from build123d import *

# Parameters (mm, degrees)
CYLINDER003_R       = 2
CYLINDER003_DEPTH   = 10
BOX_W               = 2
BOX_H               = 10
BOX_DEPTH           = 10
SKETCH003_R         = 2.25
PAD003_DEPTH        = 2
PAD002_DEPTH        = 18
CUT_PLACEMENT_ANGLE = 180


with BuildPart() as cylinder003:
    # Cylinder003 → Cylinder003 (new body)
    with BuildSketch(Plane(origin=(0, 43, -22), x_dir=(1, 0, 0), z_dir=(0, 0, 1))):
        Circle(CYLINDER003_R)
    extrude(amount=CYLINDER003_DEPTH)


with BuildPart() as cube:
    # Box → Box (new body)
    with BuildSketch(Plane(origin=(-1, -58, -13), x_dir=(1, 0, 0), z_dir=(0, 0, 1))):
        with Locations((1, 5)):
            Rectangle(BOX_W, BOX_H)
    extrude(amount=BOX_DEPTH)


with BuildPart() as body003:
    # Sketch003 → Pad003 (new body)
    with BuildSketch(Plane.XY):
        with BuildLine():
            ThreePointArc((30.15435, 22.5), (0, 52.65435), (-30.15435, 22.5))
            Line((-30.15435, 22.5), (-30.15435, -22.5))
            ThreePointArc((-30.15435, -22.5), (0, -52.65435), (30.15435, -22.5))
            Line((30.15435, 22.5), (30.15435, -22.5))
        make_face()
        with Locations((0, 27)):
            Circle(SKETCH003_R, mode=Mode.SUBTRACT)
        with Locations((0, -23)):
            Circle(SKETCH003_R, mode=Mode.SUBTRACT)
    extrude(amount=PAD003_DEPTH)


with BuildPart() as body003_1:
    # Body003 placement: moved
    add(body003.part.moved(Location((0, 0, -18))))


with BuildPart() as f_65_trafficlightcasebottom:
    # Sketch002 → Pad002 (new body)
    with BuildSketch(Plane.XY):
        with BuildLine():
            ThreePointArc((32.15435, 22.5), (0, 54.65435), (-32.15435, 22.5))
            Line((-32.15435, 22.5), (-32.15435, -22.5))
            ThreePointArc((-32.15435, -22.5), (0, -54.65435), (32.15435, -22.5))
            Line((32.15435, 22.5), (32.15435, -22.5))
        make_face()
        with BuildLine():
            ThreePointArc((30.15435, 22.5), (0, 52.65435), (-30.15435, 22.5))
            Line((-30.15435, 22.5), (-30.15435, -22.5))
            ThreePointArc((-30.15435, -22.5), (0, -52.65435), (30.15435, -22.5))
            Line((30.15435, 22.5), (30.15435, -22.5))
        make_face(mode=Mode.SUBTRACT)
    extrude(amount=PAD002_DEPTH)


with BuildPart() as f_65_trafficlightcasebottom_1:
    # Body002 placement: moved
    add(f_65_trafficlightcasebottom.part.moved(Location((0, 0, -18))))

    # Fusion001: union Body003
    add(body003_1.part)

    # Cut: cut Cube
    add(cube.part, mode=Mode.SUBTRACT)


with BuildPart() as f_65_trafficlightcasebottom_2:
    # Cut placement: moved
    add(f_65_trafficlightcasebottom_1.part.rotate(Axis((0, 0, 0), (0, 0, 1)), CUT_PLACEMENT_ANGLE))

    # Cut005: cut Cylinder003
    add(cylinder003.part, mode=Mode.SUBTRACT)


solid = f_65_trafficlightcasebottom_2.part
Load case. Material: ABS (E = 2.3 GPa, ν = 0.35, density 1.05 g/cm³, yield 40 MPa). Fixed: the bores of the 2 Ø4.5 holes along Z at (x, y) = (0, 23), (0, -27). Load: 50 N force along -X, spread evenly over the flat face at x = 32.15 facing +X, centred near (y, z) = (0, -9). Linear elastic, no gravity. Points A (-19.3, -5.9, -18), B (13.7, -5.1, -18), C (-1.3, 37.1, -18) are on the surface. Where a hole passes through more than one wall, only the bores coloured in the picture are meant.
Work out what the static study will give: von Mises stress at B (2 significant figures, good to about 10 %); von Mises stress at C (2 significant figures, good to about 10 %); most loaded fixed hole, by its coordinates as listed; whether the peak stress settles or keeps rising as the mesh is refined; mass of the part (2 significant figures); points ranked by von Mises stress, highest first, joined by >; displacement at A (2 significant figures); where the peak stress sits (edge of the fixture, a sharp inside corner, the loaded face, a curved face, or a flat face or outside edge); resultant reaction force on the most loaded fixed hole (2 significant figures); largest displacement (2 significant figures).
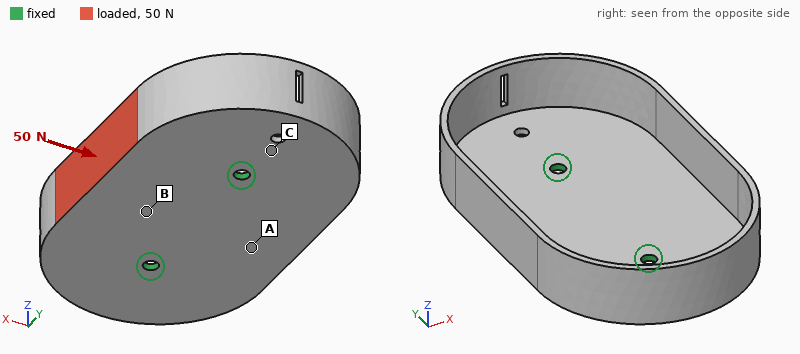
2.9 MPa
1.9 MPa
(0, 23)
keeps rising
22 g
B > C > A
0.27 mm
edge of the fixture
28 N
1.5 mm
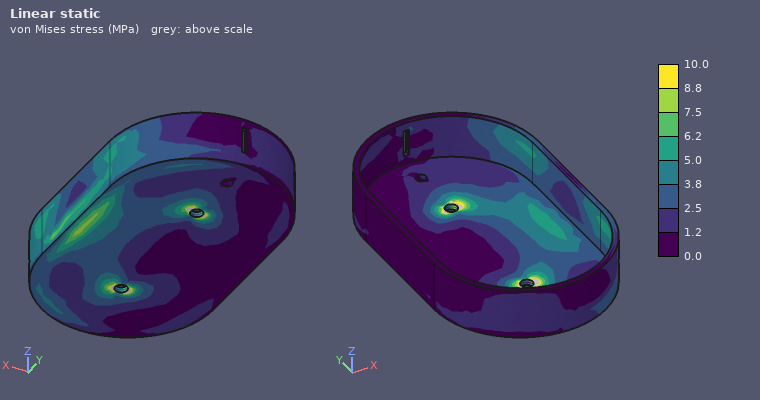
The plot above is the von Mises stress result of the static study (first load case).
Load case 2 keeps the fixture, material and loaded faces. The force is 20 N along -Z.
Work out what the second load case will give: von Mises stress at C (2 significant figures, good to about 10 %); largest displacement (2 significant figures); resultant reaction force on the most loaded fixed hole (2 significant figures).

2.8 MPa
1.4 mm
11 N
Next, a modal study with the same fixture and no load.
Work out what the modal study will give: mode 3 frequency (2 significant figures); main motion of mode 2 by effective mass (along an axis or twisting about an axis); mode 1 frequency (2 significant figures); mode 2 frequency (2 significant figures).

420 Hz
along Z
230 Hz
400 Hz
